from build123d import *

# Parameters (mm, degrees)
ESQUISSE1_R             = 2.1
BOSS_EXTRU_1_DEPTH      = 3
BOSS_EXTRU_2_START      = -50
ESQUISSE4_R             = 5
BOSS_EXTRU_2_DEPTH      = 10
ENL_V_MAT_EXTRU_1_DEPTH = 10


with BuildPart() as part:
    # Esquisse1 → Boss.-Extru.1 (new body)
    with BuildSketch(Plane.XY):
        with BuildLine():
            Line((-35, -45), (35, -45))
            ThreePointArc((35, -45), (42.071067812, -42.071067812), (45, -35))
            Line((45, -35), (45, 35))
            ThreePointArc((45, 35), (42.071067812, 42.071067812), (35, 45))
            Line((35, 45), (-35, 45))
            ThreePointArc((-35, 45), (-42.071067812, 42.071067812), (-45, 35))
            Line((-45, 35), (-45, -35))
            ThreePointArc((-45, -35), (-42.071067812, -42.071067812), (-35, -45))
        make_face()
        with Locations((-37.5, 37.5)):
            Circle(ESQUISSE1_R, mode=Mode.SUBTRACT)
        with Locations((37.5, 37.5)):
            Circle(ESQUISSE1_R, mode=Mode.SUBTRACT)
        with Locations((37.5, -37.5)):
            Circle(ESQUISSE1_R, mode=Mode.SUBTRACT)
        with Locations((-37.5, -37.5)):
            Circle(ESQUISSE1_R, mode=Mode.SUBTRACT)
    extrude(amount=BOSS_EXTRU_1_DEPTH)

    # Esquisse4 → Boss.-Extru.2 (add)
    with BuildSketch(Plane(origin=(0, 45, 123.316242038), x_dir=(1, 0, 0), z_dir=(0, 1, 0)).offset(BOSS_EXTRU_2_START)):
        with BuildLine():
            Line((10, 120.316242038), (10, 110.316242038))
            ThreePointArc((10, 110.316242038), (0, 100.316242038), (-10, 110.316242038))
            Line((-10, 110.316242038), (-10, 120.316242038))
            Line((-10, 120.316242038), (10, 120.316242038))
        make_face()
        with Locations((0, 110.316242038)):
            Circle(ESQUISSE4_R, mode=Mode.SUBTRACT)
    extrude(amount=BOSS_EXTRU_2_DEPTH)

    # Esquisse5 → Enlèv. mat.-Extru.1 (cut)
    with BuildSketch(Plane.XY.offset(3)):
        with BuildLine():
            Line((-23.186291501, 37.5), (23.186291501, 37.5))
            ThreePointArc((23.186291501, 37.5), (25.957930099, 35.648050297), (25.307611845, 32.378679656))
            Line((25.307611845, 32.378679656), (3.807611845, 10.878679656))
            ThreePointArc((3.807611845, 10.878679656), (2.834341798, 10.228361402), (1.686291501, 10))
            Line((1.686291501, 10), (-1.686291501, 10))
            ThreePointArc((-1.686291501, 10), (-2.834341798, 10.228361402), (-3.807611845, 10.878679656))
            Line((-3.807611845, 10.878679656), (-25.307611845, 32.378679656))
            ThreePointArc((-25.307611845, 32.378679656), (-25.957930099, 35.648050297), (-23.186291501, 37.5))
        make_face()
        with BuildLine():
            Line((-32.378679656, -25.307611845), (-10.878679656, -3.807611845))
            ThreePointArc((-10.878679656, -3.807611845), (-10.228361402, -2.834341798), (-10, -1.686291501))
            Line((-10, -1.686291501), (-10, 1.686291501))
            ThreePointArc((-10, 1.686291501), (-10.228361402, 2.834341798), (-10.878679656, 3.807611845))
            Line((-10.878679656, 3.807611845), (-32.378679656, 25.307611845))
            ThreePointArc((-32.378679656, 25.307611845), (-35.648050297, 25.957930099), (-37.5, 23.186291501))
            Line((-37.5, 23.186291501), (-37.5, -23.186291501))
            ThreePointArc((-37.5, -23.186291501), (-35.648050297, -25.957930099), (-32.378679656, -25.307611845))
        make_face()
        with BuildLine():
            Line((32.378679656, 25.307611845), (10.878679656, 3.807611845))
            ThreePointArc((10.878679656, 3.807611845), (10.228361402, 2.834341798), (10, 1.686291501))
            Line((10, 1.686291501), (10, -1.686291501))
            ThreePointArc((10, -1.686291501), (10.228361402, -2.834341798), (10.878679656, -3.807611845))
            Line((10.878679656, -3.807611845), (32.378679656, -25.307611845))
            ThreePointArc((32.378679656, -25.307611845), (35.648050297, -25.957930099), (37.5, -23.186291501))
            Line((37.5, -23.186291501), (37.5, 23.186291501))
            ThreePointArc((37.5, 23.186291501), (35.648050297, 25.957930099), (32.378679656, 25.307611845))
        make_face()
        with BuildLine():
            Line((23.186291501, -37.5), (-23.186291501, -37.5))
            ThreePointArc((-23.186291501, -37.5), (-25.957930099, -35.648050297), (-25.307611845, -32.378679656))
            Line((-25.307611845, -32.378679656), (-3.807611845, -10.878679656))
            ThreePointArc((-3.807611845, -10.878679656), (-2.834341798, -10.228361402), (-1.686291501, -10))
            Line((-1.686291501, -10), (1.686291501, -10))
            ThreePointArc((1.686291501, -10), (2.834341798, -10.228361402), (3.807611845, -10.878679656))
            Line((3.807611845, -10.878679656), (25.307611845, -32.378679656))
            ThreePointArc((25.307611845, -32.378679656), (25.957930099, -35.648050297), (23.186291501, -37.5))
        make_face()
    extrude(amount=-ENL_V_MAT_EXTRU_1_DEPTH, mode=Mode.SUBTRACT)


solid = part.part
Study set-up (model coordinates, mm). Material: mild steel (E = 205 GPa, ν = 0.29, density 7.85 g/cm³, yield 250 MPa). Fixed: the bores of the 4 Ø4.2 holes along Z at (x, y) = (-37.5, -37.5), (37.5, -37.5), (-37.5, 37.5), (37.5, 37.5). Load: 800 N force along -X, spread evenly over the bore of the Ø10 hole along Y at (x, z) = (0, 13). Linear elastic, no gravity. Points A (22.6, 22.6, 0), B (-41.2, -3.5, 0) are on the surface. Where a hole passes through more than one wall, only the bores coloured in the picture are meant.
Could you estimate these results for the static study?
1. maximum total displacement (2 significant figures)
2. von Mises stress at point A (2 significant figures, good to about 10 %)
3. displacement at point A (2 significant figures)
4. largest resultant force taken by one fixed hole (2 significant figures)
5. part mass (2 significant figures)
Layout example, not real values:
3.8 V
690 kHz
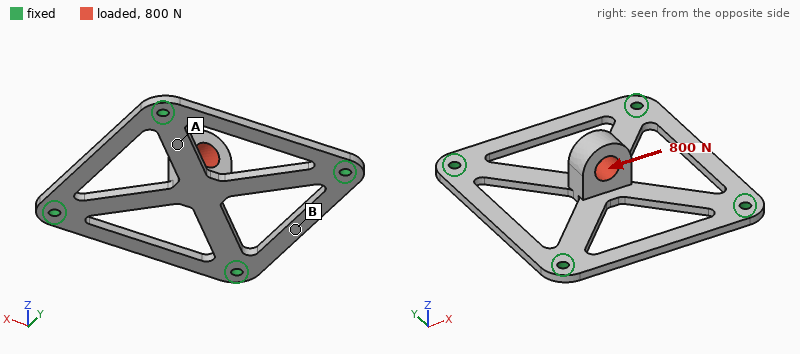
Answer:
0.12 mm
42 MPa
0.027 mm
280 N
130 g
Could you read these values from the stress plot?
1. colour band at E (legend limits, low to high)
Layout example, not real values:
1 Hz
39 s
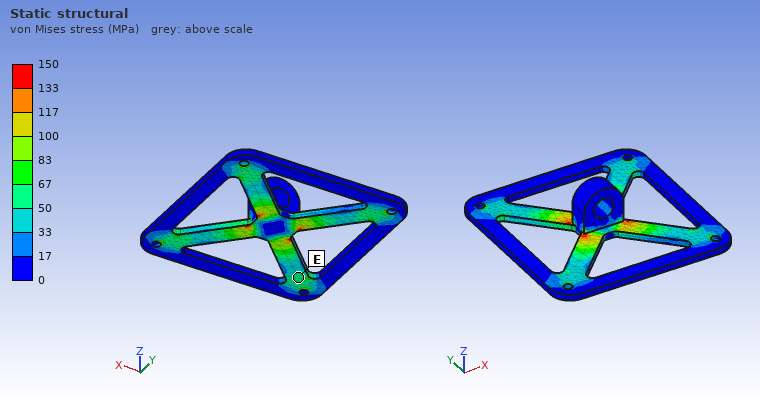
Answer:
50 to 67 MPa
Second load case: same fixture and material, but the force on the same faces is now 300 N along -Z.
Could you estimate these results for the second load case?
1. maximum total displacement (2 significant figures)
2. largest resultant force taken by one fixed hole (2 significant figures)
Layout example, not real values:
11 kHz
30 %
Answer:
0.10 mm
80 N
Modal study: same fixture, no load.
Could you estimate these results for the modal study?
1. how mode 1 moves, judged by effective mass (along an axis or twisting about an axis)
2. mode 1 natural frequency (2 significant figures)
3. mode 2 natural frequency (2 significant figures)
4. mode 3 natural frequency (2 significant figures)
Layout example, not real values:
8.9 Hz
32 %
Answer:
along Z
1300 Hz
2800 Hz
2800 Hz
